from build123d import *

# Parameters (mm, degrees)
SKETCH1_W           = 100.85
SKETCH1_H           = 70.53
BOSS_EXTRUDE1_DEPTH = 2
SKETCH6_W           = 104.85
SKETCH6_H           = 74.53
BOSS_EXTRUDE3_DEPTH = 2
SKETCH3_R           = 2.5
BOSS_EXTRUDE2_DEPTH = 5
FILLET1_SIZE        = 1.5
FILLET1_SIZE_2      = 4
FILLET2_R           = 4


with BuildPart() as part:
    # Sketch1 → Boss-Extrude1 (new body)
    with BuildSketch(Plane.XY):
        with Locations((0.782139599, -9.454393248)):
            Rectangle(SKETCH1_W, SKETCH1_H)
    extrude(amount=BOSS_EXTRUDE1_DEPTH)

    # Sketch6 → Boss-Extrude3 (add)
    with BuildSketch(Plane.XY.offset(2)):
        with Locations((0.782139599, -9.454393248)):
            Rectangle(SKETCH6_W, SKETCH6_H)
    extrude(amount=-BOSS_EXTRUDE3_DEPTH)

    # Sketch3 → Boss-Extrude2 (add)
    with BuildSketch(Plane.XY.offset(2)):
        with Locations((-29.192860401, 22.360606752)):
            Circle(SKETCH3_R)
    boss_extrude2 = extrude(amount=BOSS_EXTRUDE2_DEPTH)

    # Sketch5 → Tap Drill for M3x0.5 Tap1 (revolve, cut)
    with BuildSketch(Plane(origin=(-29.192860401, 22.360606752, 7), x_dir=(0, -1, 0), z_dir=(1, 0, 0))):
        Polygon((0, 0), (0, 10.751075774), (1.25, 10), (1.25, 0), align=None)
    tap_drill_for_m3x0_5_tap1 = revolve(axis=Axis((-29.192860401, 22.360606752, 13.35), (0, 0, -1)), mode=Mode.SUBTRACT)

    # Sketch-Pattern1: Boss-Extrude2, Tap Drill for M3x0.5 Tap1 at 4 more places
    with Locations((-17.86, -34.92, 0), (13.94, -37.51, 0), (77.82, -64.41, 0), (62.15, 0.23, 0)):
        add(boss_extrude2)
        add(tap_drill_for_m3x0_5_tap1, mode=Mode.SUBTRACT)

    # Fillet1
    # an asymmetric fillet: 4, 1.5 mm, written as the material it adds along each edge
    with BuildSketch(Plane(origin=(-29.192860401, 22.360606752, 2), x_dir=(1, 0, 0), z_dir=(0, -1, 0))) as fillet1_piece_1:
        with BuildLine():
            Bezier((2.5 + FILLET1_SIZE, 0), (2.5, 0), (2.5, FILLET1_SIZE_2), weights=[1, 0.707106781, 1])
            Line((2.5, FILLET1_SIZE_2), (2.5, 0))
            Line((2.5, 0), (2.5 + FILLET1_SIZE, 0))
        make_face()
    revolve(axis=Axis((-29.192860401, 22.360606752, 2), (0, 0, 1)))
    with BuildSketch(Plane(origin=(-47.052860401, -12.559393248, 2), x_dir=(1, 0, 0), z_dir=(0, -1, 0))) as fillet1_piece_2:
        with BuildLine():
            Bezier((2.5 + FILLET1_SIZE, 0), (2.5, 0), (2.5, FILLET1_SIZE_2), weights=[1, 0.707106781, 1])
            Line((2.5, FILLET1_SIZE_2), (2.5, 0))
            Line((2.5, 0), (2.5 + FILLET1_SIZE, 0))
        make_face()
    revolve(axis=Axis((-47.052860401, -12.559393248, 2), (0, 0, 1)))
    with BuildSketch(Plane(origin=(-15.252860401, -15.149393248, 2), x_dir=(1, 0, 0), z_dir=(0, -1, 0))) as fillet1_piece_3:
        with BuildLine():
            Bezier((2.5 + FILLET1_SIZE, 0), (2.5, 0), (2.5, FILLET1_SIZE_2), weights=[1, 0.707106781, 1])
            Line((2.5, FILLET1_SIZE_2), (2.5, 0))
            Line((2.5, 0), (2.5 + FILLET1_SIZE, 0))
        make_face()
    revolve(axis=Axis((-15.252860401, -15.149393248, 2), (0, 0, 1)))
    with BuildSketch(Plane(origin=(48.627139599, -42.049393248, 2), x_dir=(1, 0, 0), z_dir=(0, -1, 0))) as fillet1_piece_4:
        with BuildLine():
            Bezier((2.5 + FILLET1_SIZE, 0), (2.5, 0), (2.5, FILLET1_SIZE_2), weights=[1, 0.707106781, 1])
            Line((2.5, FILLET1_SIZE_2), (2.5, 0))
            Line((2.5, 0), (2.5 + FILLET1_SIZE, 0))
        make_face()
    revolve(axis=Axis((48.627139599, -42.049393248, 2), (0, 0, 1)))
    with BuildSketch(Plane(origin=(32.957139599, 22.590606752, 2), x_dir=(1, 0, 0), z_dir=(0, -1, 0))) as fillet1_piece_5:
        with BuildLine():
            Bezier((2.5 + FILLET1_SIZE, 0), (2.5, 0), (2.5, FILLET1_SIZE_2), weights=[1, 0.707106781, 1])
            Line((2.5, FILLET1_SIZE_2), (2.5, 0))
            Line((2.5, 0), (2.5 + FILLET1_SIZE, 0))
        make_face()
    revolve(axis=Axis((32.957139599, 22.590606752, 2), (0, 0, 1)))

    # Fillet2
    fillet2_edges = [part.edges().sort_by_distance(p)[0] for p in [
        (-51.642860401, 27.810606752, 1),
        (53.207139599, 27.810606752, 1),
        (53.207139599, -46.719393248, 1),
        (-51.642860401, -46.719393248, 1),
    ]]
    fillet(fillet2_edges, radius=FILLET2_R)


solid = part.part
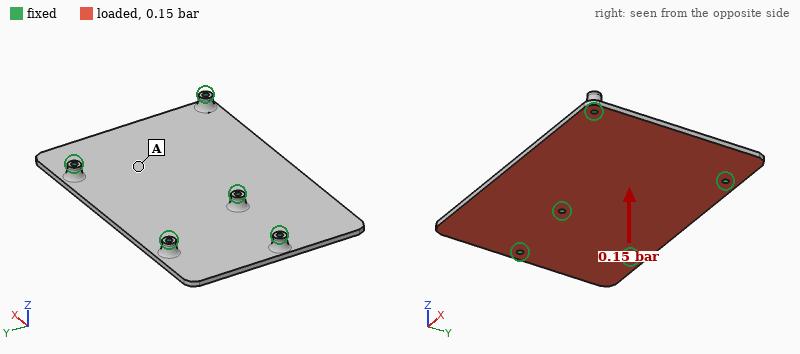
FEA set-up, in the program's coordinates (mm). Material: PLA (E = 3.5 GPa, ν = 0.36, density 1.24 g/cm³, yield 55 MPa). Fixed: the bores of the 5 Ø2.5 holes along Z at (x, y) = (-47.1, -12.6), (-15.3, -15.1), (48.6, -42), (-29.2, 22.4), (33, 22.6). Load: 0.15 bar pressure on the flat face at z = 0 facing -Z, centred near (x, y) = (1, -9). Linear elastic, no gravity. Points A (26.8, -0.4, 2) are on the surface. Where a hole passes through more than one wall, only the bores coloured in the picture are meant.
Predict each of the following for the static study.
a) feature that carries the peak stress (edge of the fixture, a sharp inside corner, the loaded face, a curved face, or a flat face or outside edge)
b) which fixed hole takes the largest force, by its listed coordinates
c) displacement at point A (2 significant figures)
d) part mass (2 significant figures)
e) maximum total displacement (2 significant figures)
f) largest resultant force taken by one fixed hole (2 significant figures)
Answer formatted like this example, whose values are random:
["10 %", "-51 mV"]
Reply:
["a curved face", "(-15.3, -15.1)", "0.28 mm", "20 g", "0.76 mm", "43 N"]
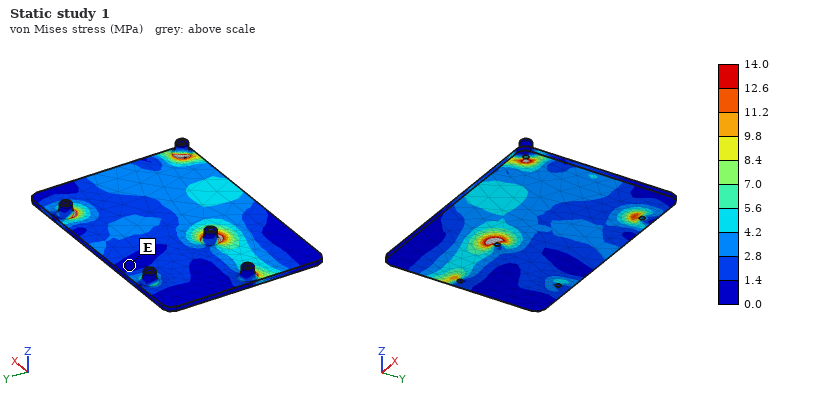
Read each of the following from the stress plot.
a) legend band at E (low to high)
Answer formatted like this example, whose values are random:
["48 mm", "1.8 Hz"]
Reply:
["0.0 to 1.4 MPa"]
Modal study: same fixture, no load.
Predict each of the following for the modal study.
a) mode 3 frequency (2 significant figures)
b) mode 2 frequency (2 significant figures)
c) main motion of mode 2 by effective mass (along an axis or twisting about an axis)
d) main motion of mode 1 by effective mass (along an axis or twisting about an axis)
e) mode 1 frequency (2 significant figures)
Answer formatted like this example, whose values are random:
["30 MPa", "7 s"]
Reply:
["830 Hz", "710 Hz", "along Z", "along Z", "560 Hz"]
